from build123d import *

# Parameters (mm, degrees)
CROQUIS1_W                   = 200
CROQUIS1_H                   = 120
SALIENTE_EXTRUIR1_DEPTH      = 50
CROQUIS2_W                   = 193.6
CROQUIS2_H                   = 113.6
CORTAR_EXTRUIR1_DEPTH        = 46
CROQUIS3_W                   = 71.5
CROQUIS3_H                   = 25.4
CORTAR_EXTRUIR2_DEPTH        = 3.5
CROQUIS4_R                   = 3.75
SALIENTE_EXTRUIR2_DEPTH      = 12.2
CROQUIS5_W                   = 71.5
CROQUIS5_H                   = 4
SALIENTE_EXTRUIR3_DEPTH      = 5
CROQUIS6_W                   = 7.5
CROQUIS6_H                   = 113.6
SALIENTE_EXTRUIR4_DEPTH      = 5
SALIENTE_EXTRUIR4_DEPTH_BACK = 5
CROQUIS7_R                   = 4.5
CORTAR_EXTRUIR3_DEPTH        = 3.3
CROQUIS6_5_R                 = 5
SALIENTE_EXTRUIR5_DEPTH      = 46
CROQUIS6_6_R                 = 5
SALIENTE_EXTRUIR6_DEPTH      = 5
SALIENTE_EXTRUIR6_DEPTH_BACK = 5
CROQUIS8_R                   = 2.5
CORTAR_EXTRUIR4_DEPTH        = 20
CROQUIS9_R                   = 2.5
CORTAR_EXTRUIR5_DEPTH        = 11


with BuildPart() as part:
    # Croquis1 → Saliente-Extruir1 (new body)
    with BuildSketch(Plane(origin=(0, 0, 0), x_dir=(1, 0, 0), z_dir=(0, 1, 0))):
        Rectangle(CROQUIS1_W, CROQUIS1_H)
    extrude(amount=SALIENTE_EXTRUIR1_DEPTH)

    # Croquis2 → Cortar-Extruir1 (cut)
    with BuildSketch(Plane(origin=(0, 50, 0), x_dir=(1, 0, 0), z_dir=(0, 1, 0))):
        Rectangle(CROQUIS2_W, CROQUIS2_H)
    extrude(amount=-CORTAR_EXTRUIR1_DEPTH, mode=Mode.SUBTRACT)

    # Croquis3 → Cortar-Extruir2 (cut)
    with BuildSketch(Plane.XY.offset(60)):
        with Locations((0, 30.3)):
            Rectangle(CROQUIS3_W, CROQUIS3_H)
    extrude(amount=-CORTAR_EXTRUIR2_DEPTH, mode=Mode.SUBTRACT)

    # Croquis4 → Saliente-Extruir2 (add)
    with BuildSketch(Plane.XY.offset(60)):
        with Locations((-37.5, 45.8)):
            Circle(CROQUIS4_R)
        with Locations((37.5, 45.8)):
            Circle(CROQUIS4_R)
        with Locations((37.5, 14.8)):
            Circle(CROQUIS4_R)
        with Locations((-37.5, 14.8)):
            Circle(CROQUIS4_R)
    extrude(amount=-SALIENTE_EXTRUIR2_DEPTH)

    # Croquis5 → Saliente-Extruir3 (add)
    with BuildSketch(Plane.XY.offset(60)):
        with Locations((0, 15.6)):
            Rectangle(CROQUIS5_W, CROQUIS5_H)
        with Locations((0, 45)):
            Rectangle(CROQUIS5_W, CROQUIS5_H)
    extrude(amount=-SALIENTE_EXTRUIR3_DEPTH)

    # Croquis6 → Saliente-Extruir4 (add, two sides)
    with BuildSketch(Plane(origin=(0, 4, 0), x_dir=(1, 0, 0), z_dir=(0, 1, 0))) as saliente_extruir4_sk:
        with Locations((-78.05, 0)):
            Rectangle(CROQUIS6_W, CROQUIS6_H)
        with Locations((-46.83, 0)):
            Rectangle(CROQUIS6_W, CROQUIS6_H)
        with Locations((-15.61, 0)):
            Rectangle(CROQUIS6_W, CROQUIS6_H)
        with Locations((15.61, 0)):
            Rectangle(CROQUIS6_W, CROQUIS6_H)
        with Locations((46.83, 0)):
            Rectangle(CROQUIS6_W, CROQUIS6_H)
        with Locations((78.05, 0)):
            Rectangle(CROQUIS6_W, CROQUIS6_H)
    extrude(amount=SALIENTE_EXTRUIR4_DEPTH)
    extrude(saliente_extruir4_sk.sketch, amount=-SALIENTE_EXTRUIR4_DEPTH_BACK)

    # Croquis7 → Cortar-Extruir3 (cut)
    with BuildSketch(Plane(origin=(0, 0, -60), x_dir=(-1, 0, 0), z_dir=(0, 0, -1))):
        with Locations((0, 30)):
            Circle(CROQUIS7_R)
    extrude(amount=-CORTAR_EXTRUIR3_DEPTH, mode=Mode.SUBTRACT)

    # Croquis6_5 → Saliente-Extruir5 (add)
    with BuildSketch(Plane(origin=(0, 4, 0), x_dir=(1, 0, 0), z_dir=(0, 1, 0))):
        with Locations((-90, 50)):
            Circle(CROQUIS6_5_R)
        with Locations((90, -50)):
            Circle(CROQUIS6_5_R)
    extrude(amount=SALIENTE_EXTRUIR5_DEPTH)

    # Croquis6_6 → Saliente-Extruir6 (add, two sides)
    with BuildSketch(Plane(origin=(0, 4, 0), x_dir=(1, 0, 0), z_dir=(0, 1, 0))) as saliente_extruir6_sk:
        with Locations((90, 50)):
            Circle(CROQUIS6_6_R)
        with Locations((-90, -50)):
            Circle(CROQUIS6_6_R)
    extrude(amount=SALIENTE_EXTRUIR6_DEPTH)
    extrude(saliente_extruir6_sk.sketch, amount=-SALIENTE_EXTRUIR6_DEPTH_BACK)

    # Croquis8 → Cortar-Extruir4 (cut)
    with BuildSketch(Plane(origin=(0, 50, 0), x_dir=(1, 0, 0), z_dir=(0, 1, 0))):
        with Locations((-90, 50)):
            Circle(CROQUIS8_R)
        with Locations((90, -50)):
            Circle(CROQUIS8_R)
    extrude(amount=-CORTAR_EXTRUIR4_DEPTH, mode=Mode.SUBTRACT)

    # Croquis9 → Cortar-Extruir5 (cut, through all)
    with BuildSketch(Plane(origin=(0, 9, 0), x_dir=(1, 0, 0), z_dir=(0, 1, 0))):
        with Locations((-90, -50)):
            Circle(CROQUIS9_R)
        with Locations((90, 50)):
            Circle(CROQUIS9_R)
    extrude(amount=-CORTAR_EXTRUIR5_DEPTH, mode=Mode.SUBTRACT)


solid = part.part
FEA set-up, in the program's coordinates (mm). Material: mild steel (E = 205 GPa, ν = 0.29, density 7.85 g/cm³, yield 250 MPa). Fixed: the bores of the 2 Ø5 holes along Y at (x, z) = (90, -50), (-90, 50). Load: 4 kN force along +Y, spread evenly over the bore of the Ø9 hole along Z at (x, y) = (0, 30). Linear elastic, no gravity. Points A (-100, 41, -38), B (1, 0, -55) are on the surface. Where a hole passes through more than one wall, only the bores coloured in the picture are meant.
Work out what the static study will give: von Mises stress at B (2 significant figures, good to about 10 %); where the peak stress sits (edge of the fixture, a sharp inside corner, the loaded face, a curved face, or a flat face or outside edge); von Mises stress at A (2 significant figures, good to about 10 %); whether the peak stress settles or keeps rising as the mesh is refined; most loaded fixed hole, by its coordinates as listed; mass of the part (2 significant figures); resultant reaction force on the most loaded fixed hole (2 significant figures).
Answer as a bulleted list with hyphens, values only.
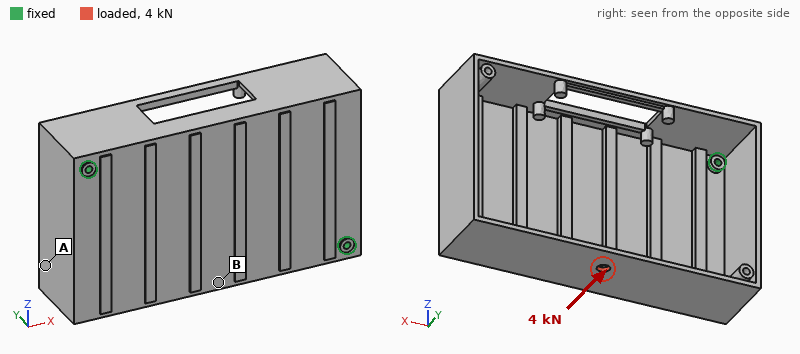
- 49 MPa
- edge of the fixture
- 27 MPa
- keeps rising
- (90, -50)
- 1.7 kg
- 2.7 kN
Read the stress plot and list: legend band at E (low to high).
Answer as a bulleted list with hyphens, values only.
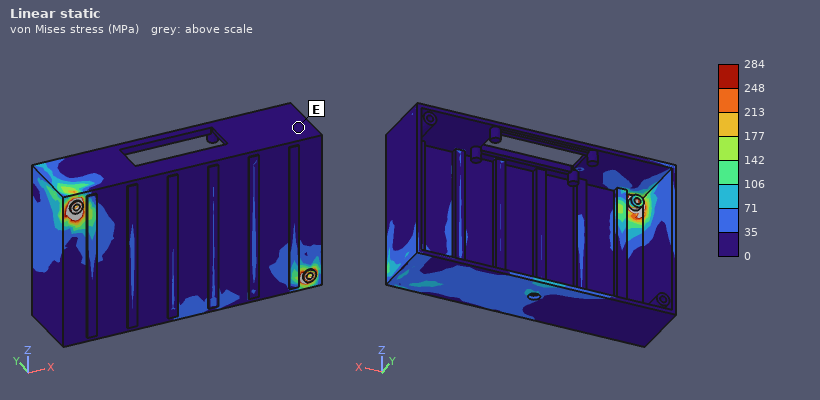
- 0 to 35 MPa
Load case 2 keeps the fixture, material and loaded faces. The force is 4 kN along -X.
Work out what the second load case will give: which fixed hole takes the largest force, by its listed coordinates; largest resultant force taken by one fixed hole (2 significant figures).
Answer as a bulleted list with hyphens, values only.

- (90, -50)
- 3.1 kN
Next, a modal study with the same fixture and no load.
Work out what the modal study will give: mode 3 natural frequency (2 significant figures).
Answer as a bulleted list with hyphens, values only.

- 1200 Hz
